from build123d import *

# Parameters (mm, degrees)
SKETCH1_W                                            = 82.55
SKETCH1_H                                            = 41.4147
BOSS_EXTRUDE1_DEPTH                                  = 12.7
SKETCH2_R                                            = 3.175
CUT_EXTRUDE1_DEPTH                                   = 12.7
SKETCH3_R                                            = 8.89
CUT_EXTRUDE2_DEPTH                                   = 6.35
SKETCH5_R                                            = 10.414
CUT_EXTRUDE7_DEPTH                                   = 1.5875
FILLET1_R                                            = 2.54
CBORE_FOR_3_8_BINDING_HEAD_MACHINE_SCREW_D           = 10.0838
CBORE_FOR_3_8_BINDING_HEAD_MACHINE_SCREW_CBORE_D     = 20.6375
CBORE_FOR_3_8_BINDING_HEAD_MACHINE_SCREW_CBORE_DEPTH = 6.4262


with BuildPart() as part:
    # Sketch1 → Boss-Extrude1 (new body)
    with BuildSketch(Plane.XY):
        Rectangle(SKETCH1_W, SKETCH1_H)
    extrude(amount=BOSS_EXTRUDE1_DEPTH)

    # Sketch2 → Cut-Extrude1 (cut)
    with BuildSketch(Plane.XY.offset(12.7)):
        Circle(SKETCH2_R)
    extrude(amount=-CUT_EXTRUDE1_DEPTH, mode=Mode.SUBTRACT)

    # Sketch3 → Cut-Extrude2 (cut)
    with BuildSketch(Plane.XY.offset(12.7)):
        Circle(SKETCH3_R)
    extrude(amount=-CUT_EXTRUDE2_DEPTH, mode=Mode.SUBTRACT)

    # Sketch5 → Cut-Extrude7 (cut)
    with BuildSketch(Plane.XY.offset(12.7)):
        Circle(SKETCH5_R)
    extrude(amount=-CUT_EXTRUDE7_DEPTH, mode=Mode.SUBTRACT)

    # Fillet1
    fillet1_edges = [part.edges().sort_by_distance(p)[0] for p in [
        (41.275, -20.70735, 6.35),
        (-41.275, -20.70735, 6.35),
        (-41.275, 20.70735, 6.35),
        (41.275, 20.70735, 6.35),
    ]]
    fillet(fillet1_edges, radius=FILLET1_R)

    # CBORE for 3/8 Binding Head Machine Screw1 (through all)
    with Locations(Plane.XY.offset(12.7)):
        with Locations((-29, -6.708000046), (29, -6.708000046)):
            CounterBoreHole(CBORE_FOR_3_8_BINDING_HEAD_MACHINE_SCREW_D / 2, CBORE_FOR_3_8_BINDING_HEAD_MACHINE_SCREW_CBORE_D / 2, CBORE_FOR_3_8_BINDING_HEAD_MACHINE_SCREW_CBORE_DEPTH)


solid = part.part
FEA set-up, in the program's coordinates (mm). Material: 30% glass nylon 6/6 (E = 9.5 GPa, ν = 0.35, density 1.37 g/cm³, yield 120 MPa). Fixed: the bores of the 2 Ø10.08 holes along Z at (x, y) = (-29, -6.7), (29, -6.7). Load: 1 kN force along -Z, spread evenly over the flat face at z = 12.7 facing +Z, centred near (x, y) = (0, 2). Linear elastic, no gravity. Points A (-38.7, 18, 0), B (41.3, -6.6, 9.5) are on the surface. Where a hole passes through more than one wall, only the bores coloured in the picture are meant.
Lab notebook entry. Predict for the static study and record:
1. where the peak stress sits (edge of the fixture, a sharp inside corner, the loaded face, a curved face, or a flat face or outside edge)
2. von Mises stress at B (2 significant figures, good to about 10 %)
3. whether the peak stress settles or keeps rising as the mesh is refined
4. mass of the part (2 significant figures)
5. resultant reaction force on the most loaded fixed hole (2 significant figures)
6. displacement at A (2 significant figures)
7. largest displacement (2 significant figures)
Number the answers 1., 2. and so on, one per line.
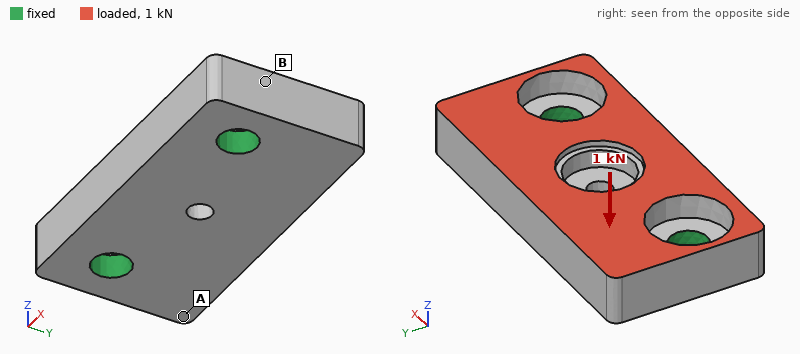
1. edge of the fixture
2. 4.9 MPa
3. keeps rising
4. 49 g
5. 520 N
6. 47 µm
7. 78 µm
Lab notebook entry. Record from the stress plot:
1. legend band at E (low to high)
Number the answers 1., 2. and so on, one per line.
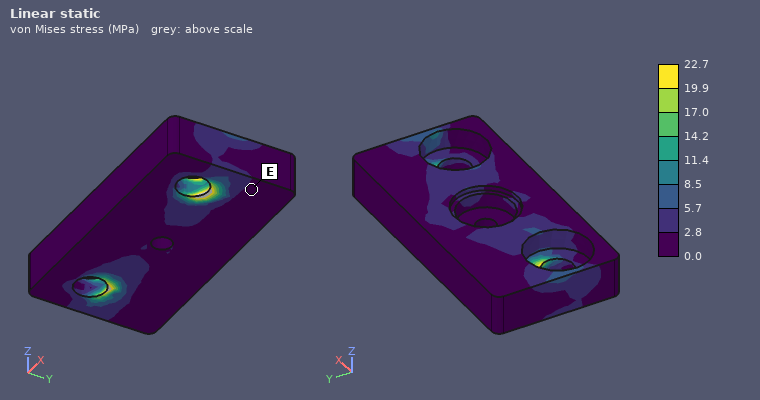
1. 0.0 to 2.8 MPa
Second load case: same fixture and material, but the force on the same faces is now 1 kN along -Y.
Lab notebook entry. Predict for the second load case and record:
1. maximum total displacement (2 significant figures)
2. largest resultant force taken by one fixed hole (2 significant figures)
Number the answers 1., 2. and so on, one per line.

1. 71 µm
2. 500 N
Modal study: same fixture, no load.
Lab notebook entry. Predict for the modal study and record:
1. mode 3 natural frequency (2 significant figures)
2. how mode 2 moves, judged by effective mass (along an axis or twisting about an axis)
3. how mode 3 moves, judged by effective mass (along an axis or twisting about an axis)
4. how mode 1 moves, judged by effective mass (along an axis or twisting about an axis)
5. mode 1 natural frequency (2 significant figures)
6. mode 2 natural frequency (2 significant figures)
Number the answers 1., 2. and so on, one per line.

1. 6200 Hz
2. twisting about Y
3. along Z
4. along Z
5. 3200 Hz
6. 5500 Hz
